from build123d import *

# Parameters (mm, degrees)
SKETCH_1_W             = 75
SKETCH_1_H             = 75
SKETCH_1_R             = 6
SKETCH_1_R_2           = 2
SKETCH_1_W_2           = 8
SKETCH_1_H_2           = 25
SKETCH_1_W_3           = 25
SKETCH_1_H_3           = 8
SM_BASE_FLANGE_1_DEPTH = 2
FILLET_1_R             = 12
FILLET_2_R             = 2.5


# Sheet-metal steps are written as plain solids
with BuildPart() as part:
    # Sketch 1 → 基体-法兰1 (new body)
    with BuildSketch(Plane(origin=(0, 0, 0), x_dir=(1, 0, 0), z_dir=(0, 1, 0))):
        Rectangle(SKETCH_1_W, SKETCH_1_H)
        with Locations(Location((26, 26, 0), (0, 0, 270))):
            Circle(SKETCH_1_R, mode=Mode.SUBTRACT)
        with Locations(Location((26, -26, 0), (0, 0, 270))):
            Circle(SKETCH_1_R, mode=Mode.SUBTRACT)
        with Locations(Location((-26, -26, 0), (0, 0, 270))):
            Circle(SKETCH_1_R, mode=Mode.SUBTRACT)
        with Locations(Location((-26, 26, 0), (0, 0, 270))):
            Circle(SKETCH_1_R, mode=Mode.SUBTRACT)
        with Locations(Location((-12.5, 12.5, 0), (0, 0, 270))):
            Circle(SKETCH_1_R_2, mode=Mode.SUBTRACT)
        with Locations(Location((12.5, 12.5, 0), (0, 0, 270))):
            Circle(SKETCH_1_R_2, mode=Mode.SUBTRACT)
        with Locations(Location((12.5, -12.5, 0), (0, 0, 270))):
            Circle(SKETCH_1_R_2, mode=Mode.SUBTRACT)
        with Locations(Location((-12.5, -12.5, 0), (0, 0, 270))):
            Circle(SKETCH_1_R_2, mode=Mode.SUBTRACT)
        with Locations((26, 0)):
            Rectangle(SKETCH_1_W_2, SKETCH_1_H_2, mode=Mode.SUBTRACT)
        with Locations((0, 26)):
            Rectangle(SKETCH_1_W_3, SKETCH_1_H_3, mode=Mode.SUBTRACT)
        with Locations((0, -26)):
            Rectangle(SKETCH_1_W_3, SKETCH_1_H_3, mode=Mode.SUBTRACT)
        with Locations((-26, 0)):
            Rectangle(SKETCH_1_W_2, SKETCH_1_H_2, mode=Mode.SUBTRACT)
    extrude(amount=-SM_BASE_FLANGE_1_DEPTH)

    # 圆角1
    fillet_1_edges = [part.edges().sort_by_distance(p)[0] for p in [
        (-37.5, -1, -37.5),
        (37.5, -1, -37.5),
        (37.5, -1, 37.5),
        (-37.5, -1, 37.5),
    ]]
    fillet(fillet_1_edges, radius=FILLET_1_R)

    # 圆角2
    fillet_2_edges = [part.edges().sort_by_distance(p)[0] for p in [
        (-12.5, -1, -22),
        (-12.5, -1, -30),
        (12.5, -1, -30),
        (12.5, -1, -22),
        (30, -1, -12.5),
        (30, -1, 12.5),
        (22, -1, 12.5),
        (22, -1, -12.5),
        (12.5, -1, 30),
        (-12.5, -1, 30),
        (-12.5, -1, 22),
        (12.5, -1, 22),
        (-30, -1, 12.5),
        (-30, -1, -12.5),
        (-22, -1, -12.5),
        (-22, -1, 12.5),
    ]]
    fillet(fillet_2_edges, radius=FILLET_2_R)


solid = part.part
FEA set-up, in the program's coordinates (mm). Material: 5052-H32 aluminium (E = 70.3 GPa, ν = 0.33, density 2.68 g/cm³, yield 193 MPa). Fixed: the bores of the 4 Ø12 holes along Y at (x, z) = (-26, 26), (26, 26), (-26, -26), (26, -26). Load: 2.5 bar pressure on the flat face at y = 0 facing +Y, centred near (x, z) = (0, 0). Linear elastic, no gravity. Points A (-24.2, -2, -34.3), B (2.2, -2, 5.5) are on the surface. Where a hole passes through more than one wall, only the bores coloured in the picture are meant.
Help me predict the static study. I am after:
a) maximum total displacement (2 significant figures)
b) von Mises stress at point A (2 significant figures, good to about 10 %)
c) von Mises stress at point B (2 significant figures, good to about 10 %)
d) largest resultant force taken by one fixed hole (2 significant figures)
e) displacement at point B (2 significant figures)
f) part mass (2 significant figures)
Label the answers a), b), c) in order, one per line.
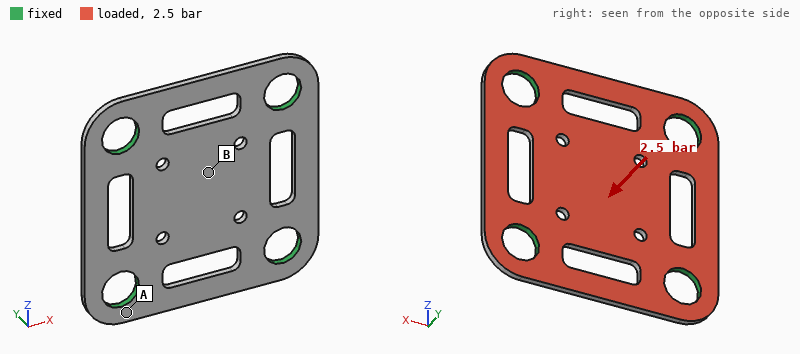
a) 0.12 mm
b) 11 MPa
c) 34 MPa
d) 260 N
e) 0.11 mm
f) 23 g
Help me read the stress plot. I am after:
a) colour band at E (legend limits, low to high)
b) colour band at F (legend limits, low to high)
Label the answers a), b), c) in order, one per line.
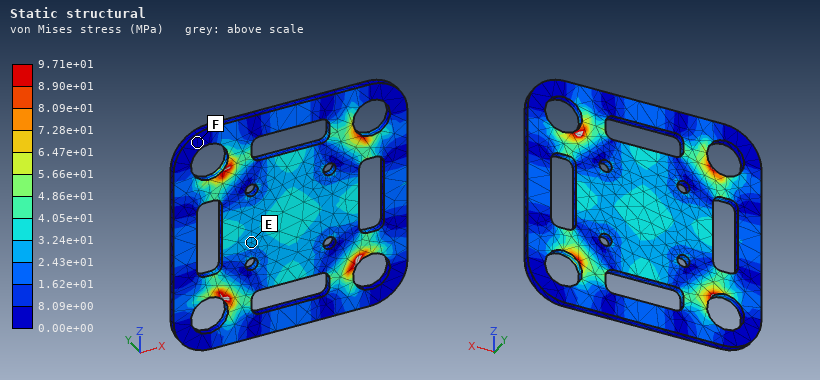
a) 2.43e+01 to 3.24e+01 MPa
b) 0.00e+00 to 8.09e+00 MPa
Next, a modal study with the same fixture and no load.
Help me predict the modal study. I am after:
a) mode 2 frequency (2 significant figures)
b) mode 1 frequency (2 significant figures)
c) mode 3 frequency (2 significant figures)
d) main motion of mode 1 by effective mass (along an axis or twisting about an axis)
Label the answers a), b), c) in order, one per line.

a) 6300 Hz
b) 3800 Hz
c) 6400 Hz
d) along Y
